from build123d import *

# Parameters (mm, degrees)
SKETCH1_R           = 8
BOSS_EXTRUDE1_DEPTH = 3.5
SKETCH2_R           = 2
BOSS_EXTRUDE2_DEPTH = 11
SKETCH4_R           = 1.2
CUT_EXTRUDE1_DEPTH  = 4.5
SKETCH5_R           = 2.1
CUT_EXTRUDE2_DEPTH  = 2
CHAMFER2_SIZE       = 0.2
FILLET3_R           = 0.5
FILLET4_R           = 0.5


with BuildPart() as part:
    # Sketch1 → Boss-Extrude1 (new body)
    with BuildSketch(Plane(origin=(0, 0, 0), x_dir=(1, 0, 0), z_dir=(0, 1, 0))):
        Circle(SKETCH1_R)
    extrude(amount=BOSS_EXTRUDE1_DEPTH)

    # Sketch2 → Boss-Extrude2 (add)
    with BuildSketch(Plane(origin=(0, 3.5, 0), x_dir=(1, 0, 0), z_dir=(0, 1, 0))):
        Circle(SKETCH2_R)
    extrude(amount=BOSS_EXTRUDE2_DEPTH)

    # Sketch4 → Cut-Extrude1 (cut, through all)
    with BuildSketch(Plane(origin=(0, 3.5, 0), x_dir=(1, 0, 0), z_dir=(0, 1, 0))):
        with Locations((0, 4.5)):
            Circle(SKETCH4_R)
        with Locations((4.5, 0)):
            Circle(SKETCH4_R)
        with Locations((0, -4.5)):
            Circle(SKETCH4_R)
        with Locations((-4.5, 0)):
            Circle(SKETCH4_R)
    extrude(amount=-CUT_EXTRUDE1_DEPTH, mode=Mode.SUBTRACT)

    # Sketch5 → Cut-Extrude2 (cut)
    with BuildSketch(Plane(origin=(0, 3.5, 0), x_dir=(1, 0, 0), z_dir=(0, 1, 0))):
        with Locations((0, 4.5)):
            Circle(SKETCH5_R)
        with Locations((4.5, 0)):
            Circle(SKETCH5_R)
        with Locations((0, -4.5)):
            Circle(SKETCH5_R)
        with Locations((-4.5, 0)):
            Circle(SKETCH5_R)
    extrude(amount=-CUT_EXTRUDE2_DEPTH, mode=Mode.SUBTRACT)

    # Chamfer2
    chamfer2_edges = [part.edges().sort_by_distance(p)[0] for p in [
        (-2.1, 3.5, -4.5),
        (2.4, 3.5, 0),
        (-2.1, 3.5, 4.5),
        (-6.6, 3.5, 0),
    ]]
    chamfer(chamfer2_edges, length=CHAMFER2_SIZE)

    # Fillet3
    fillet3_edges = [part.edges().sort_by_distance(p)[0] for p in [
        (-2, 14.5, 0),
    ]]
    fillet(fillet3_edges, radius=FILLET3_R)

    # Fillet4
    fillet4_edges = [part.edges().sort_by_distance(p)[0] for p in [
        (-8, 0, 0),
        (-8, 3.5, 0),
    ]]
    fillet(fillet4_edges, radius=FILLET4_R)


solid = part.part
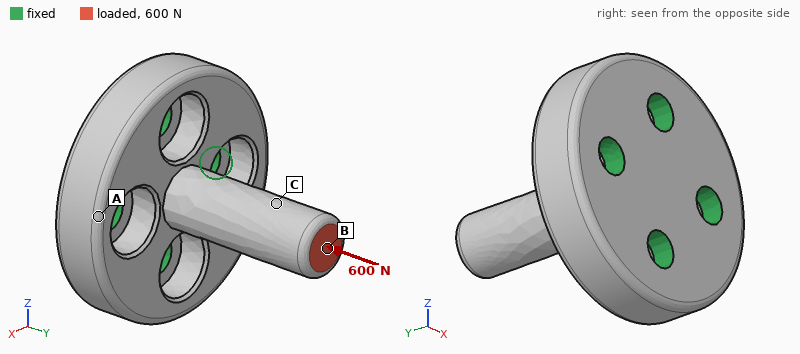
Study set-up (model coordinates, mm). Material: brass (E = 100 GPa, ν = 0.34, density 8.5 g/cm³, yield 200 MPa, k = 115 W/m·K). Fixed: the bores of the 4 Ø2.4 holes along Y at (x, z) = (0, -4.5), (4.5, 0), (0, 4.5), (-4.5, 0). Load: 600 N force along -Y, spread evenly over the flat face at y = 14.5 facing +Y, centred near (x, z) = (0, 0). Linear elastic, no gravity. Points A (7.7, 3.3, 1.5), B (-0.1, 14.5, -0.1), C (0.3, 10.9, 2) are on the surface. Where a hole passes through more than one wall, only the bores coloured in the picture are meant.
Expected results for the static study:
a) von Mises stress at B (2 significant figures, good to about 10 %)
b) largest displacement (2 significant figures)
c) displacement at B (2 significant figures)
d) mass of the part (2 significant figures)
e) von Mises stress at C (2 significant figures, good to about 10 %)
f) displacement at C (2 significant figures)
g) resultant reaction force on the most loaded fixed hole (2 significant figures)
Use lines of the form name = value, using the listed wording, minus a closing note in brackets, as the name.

von Mises stress at B = 42 MPa
largest displacement = 7.5 µm
displacement at B = 7.5 µm
mass of the part = 5.9 g
von Mises stress at C = 48 MPa
displacement at C = 5.3 µm
resultant reaction force on the most loaded fixed hole = 170 N
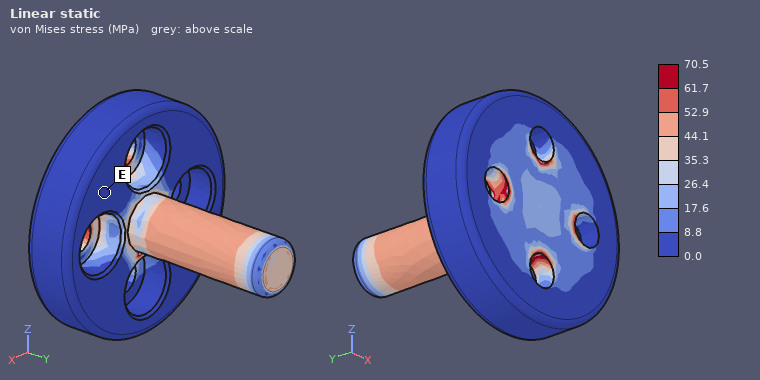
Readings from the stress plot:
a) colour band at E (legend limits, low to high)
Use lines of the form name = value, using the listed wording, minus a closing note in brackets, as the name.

colour band at E = 0.0 to 8.8 MPa
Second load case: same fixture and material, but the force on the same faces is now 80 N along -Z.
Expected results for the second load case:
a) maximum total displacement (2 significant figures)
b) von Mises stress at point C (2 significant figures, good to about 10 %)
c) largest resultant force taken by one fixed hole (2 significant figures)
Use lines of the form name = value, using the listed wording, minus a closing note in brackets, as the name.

maximum total displacement = 41 µm
von Mises stress at point C = 45 MPa
largest resultant force taken by one fixed hole = 120 N
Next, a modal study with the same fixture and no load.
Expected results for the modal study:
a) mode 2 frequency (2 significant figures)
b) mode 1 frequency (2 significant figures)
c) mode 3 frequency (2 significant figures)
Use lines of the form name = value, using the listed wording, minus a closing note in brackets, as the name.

mode 2 frequency = 12 kHz
mode 1 frequency = 12 kHz
mode 3 frequency = 45 kHz
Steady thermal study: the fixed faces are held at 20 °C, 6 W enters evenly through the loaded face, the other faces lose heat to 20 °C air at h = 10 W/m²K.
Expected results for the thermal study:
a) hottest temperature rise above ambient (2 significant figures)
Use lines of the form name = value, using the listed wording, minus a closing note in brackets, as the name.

hottest temperature rise above ambient = 55 K
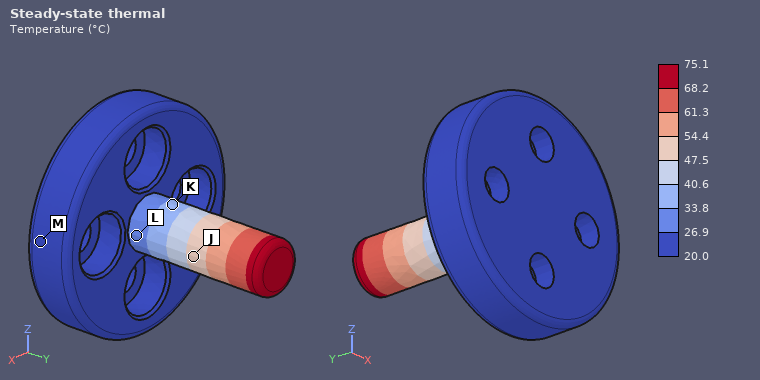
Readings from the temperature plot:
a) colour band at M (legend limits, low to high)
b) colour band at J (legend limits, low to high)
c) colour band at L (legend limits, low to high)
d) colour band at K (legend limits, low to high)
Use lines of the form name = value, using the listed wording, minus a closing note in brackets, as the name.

colour band at M = 20.0 to 26.9 °C
colour band at J = 47.5 to 54.4 °C
colour band at L = 26.9 to 33.8 °C
colour band at K = 33.8 to 40.6 °C
